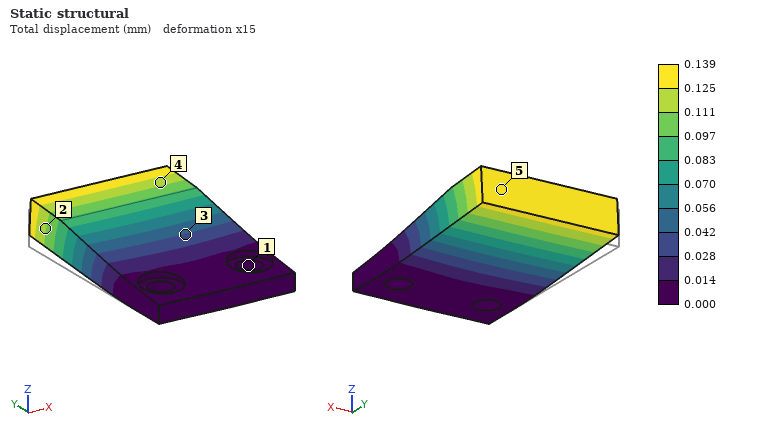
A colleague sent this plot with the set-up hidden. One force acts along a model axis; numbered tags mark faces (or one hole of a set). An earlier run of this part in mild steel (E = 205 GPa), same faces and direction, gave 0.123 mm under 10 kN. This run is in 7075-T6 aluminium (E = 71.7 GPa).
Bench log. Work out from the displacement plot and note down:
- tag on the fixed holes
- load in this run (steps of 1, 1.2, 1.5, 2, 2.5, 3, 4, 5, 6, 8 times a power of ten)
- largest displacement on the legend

1
4 kN
0.139 mm
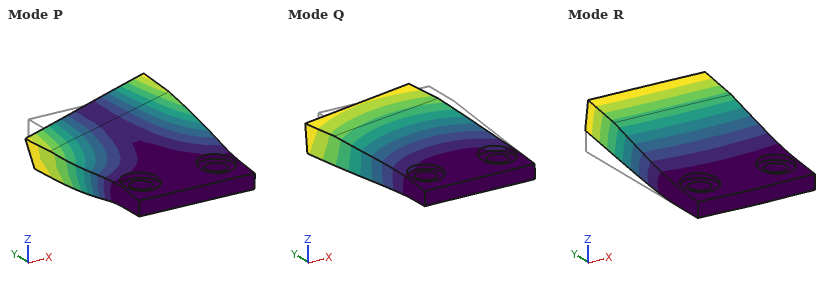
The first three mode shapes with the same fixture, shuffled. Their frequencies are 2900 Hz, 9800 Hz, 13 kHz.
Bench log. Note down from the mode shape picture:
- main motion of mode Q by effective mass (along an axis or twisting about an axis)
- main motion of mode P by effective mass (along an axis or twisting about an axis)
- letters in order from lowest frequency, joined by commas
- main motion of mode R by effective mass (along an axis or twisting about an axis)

along X
twisting about Y
R, P, Q
along Z
